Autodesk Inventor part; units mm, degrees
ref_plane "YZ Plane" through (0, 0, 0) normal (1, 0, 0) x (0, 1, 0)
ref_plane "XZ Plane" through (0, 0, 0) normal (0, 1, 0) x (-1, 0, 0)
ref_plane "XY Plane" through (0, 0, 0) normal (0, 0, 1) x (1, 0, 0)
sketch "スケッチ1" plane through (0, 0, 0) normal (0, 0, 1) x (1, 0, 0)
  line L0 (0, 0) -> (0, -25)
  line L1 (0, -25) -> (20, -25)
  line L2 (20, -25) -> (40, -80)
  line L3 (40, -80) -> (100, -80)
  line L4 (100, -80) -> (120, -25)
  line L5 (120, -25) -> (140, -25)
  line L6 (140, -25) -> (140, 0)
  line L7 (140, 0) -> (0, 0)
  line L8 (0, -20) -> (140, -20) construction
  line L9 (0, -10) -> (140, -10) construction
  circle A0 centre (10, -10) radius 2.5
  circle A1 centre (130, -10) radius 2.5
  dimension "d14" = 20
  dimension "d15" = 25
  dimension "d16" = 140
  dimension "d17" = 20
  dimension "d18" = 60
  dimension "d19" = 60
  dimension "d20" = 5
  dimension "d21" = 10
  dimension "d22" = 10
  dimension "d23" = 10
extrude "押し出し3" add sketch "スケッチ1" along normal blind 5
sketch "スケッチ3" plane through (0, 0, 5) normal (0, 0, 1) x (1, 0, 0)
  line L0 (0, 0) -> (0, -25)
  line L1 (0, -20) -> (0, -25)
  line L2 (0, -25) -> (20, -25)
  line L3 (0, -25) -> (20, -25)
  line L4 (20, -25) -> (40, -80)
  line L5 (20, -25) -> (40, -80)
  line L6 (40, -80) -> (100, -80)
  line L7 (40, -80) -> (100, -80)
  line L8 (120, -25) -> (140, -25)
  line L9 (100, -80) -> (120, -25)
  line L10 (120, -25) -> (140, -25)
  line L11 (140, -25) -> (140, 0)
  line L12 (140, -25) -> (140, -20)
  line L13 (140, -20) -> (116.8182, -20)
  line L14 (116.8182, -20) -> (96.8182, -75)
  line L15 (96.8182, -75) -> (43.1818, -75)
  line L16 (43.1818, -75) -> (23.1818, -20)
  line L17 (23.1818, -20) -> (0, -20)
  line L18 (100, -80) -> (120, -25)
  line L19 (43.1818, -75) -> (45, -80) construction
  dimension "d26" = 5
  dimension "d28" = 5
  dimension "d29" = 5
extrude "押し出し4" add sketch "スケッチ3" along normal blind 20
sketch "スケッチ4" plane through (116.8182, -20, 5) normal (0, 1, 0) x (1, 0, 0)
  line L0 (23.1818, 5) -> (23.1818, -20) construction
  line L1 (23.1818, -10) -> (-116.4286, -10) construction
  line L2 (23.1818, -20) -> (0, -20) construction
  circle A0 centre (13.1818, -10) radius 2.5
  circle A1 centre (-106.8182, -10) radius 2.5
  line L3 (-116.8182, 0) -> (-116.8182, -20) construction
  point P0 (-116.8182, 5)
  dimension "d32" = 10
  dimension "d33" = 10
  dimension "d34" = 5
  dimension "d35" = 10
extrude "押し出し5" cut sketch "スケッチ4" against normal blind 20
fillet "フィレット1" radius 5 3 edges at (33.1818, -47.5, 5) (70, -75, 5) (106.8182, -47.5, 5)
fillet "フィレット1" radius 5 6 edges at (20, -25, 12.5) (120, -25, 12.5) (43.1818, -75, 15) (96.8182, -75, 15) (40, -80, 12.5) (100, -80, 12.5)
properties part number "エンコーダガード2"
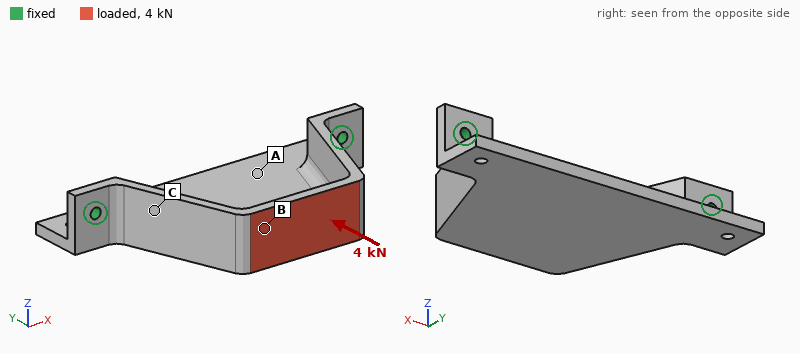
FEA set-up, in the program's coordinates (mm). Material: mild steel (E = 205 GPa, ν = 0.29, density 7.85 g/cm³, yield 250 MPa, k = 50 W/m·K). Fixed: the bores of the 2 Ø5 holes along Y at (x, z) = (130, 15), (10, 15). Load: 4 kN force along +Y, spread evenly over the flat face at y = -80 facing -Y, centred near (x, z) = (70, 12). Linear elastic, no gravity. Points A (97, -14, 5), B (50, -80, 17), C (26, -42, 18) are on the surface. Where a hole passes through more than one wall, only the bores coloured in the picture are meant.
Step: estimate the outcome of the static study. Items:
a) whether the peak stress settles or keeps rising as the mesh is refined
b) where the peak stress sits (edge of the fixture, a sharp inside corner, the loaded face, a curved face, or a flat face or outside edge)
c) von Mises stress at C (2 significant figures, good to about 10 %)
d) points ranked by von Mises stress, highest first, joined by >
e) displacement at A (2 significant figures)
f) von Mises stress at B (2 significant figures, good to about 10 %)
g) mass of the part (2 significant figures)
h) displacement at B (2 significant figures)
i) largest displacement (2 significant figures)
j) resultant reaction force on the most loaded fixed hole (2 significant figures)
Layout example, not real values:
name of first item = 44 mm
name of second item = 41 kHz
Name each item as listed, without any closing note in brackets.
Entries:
whether the peak stress settles or keeps rising as the mesh is refined = keeps rising
where the peak stress sits = edge of the fixture
von Mises stress at C = 26 MPa
points ranked by von Mises stress, highest first, joined by > = B > C > A
displacement at A = 11 µm
von Mises stress at B = 48 MPa
mass of the part = 480 g
displacement at B = 23 µm
largest displacement = 45 µm
resultant reaction force on the most loaded fixed hole = 2.1 kN
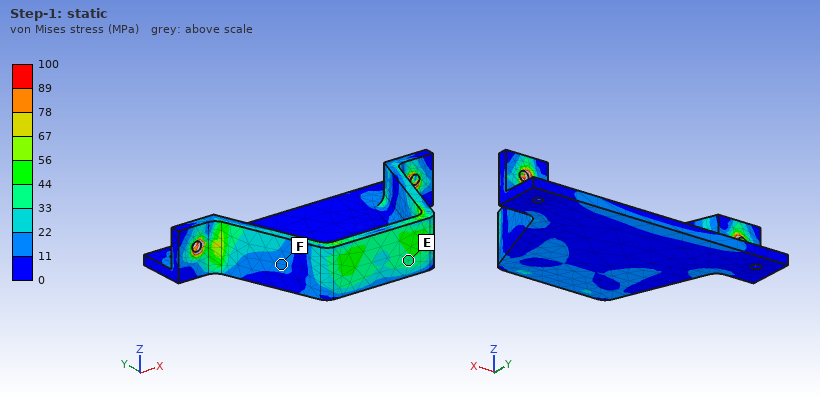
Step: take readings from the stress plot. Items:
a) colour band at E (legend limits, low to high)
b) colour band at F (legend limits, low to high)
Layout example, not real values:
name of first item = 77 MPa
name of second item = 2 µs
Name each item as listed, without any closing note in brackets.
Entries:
colour band at E = 33 to 44 MPa
colour band at F = 11 to 22 MPa
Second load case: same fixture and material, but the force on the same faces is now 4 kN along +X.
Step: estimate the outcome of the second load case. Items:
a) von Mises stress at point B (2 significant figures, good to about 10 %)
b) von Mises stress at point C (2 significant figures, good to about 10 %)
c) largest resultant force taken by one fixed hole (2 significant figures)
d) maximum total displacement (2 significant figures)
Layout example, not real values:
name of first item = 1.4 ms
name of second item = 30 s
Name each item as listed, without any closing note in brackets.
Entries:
von Mises stress at point B = 44 MPa
von Mises stress at point C = 54 MPa
largest resultant force taken by one fixed hole = 2.8 kN
maximum total displacement = 0.12 mm
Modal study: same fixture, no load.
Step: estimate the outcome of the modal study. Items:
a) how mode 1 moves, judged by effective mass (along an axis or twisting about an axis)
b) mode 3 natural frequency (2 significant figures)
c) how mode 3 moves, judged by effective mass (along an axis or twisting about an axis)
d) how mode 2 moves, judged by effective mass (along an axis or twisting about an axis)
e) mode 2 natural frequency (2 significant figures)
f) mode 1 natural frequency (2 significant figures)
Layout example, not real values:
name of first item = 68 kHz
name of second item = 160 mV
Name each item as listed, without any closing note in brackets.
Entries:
how mode 1 moves, judged by effective mass = along Z
mode 3 natural frequency = 2600 Hz
how mode 3 moves, judged by effective mass = along Z
how mode 2 moves, judged by effective mass = along X
mode 2 natural frequency = 2400 Hz
mode 1 natural frequency = 1000 Hz
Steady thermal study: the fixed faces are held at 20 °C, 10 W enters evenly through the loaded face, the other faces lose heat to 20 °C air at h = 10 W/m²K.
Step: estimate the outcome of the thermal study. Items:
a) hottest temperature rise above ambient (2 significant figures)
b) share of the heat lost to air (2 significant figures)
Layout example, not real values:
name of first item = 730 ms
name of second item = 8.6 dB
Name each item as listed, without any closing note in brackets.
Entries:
hottest temperature rise above ambient = 30 K
share of the heat lost to air = 33 %
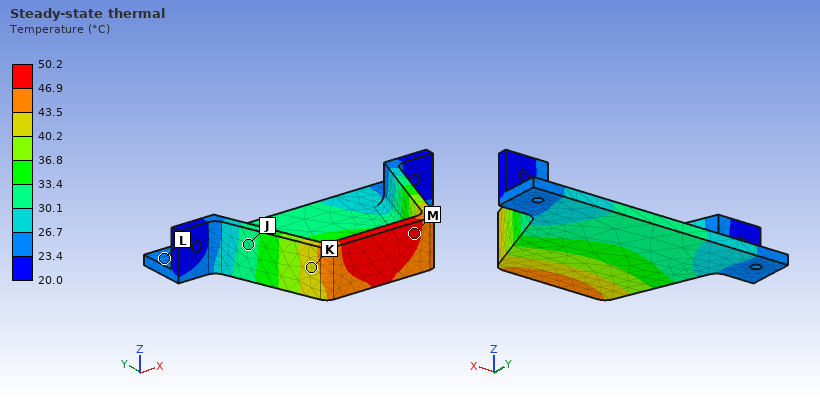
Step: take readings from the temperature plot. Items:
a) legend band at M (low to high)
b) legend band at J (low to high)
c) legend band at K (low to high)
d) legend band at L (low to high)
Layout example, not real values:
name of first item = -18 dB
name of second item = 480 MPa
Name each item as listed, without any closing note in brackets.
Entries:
legend band at M = 46.9 to 50.2 °C
legend band at J = 30.1 to 33.4 °C
legend band at K = 40.2 to 43.5 °C
legend band at L = 23.4 to 26.7 °C
